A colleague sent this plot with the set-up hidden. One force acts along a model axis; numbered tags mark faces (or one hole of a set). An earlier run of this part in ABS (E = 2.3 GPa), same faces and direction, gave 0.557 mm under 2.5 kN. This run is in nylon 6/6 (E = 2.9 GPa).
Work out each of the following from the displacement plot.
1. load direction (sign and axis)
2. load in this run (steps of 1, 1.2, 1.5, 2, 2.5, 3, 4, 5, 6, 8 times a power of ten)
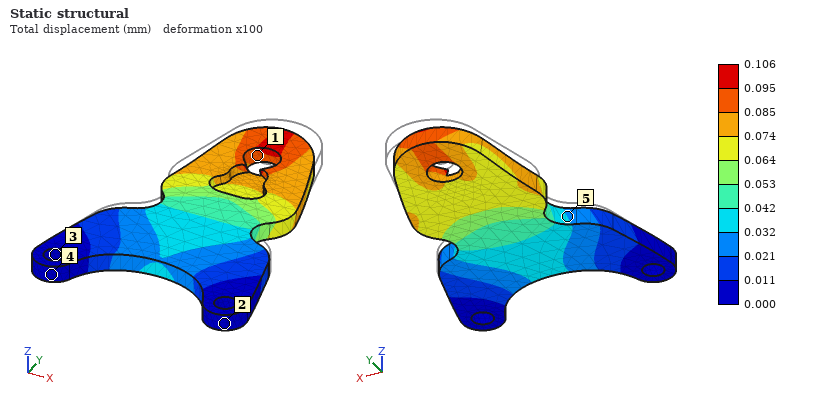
-Y
600 N
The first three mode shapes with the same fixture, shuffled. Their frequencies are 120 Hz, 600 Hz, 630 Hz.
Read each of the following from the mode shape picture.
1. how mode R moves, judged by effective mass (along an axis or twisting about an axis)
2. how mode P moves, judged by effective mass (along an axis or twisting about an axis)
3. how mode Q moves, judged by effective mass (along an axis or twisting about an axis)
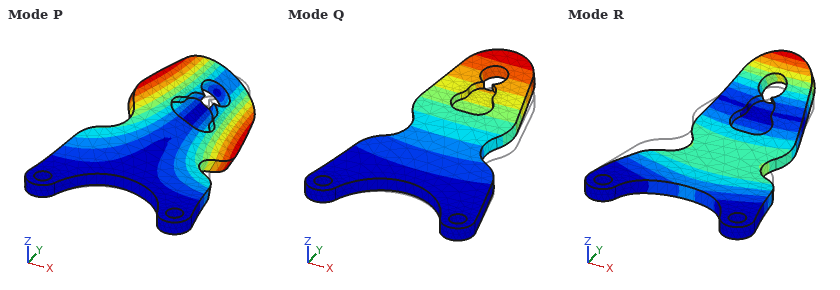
along Z
twisting about Y
along Z
